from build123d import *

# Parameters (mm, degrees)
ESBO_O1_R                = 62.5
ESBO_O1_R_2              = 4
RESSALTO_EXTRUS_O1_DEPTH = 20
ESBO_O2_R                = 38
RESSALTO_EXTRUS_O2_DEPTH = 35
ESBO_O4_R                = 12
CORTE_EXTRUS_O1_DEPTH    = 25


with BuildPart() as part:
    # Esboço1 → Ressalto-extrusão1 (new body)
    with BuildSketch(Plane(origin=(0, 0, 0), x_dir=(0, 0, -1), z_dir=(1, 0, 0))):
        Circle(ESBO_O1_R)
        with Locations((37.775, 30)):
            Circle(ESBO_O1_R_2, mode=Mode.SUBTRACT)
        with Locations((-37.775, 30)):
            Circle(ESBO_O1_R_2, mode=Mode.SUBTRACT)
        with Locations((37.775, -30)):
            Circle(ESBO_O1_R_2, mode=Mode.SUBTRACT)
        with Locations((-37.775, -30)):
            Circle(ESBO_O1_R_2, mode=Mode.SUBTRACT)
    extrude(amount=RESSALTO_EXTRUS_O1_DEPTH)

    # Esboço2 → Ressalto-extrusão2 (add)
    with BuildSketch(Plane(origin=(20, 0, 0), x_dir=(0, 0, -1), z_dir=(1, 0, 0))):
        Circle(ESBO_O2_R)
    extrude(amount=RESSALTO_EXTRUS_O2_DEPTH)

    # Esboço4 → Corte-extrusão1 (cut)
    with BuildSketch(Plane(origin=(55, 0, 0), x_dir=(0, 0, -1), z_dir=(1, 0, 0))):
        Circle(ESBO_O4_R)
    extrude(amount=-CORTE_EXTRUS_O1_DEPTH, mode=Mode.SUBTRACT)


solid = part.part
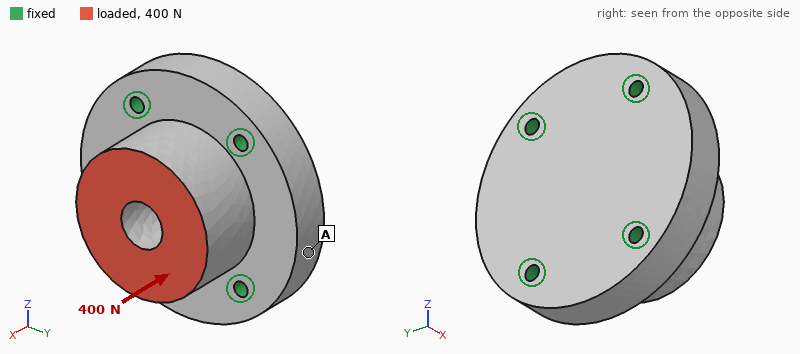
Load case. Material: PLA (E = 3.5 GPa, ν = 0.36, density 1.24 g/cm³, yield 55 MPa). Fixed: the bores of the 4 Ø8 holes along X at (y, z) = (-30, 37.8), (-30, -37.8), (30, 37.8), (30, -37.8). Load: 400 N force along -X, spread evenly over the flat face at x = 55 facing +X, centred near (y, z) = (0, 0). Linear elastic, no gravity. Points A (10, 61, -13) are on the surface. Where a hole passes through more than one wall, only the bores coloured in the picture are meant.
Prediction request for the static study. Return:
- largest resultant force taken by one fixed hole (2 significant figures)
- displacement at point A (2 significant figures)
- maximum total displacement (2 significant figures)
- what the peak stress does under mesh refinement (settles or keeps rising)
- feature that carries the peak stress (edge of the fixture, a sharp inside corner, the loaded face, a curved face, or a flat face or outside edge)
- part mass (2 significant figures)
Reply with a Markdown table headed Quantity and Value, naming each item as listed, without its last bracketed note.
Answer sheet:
| Quantity | Value |
|---|---|
| largest resultant force taken by one fixed hole | 100 N |
| displacement at point A | 2.2 µm |
| maximum total displacement | 3.9 µm |
| what the peak stress does under mesh refinement | keeps rising |
| feature that carries the peak stress | edge of the fixture |
| part mass | 480 g |
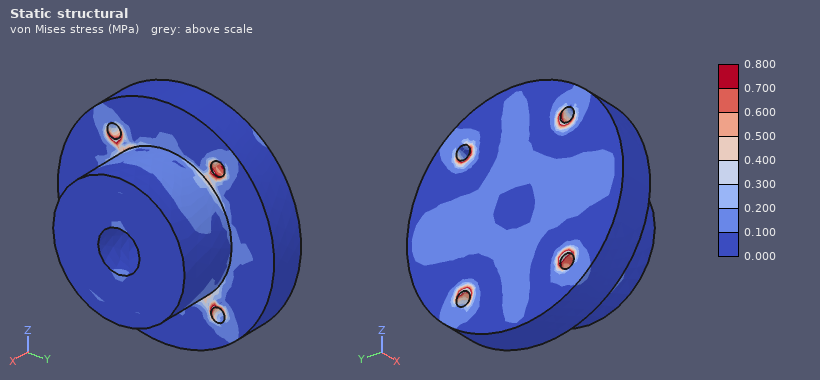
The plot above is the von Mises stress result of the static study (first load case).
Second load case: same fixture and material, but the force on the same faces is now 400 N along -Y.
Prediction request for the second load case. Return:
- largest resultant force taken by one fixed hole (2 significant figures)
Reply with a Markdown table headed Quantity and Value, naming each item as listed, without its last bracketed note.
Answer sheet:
| Quantity | Value |
|---|---|
| largest resultant force taken by one fixed hole | 170 N |
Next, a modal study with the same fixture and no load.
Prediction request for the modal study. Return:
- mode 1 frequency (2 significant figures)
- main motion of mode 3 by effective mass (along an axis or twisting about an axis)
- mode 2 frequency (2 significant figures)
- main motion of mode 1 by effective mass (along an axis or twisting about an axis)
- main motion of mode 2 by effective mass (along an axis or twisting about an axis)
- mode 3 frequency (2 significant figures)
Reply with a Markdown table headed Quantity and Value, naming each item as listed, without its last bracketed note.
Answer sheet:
| Quantity | Value |
|---|---|
| mode 1 frequency | 2600 Hz |
| main motion of mode 3 by effective mass | along Z |
| mode 2 frequency | 3000 Hz |
| main motion of mode 1 by effective mass | along Y |
| main motion of mode 2 by effective mass | along X |
| mode 3 frequency | 3300 Hz |
